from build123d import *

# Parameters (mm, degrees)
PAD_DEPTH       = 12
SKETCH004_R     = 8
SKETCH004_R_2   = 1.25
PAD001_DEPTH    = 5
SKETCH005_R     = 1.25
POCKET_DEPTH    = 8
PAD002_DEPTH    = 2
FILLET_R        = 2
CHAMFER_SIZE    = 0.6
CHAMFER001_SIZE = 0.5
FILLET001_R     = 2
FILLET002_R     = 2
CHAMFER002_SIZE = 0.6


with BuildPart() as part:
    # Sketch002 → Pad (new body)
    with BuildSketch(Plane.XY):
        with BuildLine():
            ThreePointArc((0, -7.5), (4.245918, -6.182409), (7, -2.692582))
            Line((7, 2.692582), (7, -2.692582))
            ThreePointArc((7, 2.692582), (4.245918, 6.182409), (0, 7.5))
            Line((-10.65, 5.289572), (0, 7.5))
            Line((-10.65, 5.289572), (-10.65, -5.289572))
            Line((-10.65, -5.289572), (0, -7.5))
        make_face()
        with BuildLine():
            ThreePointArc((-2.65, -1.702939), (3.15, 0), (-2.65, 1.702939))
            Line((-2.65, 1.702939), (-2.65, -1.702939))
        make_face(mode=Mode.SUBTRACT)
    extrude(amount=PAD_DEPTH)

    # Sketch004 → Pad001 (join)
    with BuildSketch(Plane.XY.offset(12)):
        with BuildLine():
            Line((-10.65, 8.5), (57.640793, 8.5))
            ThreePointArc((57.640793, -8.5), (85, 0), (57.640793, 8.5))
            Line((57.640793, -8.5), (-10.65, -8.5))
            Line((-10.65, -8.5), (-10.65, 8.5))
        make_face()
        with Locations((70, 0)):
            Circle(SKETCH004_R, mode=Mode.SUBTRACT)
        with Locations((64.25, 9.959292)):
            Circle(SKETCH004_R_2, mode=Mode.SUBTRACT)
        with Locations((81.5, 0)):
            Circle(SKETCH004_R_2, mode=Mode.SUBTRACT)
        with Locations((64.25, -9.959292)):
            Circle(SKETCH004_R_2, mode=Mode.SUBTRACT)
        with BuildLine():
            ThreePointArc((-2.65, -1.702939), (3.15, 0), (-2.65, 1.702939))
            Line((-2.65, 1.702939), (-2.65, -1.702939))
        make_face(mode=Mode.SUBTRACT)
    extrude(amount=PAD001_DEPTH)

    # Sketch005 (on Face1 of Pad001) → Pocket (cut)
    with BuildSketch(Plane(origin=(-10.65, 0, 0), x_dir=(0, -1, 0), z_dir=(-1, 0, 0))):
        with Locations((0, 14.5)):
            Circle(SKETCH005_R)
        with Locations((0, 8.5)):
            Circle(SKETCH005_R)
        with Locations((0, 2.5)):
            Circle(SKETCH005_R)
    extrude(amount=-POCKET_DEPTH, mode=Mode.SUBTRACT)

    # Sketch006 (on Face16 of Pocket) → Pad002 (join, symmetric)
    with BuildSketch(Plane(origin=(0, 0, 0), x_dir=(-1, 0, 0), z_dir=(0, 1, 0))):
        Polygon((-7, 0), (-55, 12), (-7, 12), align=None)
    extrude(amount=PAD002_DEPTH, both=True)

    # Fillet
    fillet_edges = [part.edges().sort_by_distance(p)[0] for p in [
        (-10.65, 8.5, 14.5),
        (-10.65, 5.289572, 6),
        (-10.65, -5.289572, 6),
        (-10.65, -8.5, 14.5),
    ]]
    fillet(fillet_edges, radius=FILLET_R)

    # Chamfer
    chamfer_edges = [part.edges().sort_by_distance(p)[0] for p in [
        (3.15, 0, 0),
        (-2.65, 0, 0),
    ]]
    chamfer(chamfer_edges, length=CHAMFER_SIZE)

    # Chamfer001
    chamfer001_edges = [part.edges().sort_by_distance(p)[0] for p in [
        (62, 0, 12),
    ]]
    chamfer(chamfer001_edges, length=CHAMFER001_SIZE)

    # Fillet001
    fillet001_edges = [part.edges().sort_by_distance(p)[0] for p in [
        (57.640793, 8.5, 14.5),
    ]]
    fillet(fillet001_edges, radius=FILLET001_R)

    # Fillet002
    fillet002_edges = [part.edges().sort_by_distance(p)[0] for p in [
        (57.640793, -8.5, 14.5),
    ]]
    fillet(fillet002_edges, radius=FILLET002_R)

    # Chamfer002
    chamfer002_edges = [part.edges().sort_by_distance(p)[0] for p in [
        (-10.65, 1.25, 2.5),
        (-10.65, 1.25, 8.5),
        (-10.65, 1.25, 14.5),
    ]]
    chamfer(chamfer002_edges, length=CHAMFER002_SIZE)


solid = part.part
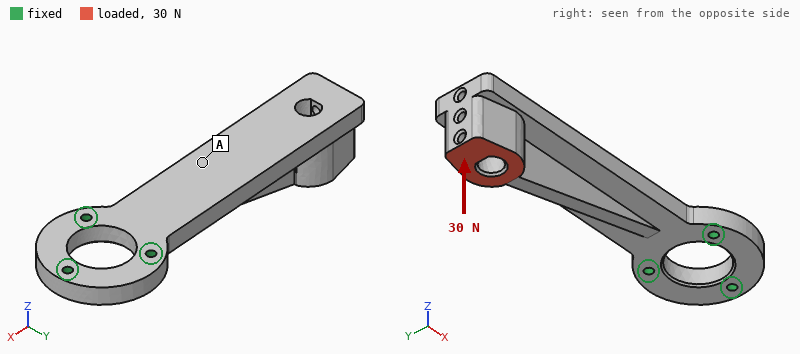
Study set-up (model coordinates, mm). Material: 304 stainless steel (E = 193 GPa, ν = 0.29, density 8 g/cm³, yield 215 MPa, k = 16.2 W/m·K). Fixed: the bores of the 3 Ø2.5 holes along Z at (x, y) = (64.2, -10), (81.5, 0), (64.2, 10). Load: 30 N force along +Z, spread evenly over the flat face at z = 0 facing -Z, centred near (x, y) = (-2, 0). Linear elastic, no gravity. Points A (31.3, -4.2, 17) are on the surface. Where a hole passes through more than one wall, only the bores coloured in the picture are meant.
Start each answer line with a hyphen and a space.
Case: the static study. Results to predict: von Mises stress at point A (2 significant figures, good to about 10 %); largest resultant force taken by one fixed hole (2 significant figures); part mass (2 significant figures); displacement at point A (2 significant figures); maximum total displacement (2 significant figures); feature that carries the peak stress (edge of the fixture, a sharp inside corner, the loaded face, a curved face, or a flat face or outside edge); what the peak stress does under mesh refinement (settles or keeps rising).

- 5.2 MPa
- 19 N
- 90 g
- 29 µm
- 85 µm
- edge of the fixture
- keeps rising
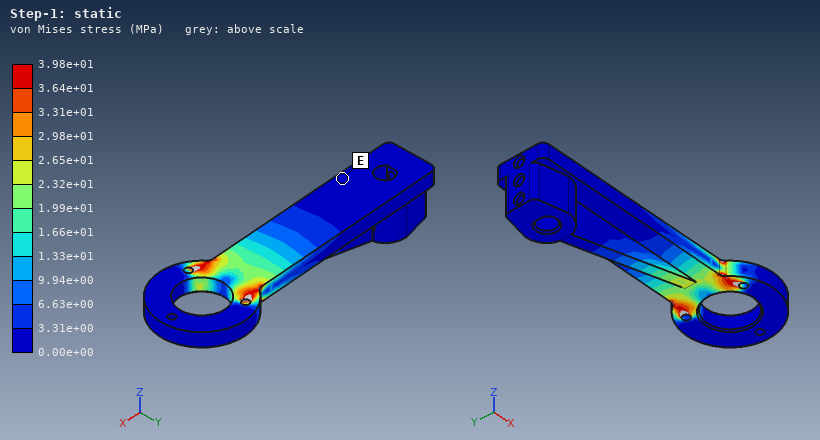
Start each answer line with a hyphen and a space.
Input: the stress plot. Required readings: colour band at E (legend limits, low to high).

- 0.00e+00 to 3.31e+00 MPa
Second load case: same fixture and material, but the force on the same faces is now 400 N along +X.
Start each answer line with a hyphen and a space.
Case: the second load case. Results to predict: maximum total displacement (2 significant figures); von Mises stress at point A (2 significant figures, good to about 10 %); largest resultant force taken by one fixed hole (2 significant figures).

- 0.30 mm
- 23 MPa
- 230 N
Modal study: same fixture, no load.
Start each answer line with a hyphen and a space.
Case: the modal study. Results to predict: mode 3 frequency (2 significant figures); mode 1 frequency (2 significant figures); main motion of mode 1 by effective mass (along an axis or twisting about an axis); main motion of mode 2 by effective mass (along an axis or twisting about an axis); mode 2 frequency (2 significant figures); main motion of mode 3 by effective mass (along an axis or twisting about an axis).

- 3900 Hz
- 520 Hz
- along Z
- along Y
- 1600 Hz
- twisting about X
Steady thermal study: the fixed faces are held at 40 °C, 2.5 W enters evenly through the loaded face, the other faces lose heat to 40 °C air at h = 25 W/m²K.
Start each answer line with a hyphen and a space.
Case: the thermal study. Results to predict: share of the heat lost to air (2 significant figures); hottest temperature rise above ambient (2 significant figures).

- 83 %
- 36 K
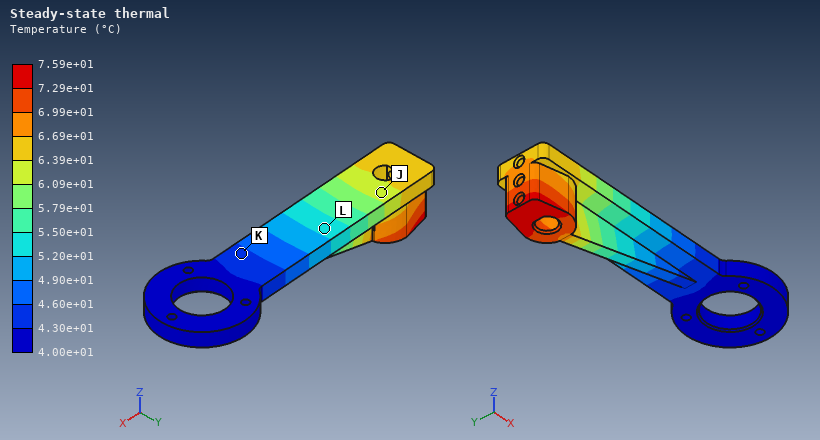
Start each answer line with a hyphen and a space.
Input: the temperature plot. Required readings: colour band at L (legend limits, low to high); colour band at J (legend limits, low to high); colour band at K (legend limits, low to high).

- 5.20e+01 to 5.50e+01 °C
- 6.09e+01 to 6.39e+01 °C
- 4.30e+01 to 4.60e+01 °C
